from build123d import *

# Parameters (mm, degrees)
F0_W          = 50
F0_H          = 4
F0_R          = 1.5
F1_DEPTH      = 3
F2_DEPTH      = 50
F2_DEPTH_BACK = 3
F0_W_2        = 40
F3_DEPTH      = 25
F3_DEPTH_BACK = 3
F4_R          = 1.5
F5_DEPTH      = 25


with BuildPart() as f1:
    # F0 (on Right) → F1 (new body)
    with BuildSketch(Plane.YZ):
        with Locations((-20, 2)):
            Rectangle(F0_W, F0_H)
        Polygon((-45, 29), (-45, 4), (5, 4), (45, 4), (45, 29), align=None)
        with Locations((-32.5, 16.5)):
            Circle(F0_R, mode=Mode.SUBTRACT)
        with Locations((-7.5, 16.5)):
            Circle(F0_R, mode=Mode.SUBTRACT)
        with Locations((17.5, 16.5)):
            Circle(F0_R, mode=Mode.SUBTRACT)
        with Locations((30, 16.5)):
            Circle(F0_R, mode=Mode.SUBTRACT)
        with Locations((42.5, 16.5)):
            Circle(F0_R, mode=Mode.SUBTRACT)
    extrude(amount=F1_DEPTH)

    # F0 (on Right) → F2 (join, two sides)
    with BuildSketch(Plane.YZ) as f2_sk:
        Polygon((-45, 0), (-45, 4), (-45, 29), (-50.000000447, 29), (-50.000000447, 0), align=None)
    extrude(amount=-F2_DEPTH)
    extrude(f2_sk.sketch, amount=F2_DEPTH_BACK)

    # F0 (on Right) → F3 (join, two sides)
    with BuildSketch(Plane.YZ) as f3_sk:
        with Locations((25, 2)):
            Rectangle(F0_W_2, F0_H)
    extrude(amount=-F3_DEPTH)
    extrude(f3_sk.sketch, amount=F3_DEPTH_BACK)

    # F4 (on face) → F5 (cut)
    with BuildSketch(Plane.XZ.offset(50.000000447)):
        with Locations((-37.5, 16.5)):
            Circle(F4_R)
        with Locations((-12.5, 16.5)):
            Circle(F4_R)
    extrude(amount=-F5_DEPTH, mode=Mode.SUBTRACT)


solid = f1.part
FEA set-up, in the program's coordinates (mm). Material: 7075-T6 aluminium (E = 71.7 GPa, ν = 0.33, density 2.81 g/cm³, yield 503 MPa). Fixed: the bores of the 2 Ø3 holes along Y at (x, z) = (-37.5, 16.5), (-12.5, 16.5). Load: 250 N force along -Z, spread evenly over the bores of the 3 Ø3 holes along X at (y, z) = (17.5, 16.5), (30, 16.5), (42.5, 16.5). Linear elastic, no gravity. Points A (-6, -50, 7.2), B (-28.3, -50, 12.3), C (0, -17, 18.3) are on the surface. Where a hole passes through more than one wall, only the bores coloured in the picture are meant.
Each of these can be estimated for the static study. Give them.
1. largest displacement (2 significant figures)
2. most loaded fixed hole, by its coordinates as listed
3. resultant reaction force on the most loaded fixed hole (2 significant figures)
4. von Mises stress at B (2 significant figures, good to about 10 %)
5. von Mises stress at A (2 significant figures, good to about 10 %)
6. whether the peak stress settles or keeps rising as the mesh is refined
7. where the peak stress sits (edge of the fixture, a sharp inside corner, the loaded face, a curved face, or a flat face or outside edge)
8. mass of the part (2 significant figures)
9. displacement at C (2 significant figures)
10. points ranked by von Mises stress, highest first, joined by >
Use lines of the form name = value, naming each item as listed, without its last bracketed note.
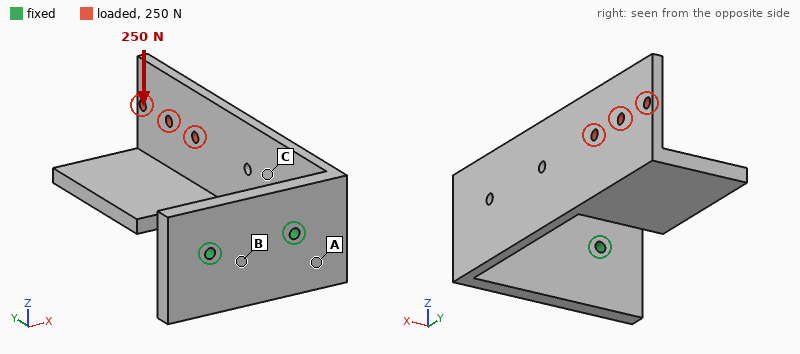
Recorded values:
largest displacement = 1.2 mm
most loaded fixed hole, by its coordinates as listed = (-12.5, 16.5)
resultant reaction force on the most loaded fixed hole = 370 N
von Mises stress at B = 28 MPa
von Mises stress at A = 85 MPa
whether the peak stress settles or keeps rising as the mesh is refined = keeps rising
where the peak stress sits = edge of the fixture
mass of the part = 54 g
displacement at C = 0.34 mm
points ranked by von Mises stress, highest first, joined by > = A > B > C
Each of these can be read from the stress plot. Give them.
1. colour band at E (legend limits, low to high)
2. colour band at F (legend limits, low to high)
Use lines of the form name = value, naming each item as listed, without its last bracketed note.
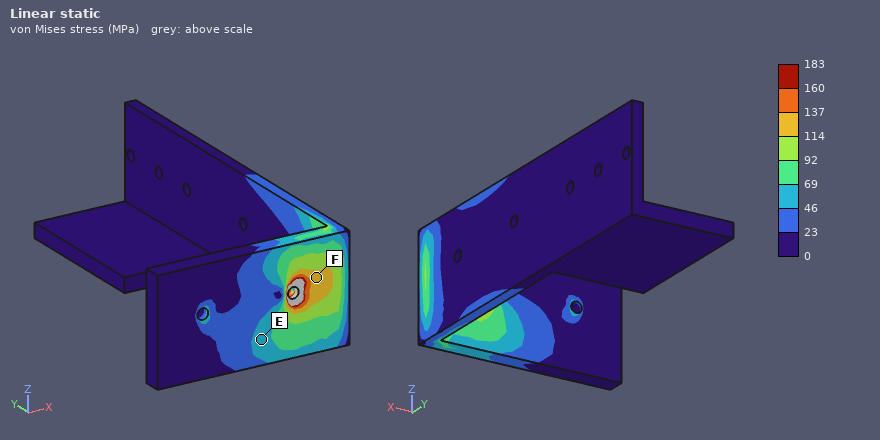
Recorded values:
colour band at E = 46 to 69 MPa
colour band at F = 114 to 137 MPa
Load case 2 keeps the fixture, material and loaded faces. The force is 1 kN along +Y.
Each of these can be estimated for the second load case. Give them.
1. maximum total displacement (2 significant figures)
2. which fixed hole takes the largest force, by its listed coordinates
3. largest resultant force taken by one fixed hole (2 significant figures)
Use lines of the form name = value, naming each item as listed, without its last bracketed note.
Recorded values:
maximum total displacement = 0.55 mm
which fixed hole takes the largest force, by its listed coordinates = (-12.5, 16.5)
largest resultant force taken by one fixed hole = 1.2 kN
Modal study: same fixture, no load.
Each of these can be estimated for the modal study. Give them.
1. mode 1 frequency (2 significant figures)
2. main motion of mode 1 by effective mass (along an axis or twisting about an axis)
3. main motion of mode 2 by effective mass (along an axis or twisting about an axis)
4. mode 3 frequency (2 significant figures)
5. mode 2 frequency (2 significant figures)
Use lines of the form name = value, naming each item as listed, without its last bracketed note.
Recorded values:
mode 1 frequency = 190 Hz
main motion of mode 1 by effective mass = along X
main motion of mode 2 by effective mass = along Z
mode 3 frequency = 1000 Hz
mode 2 frequency = 510 Hz
